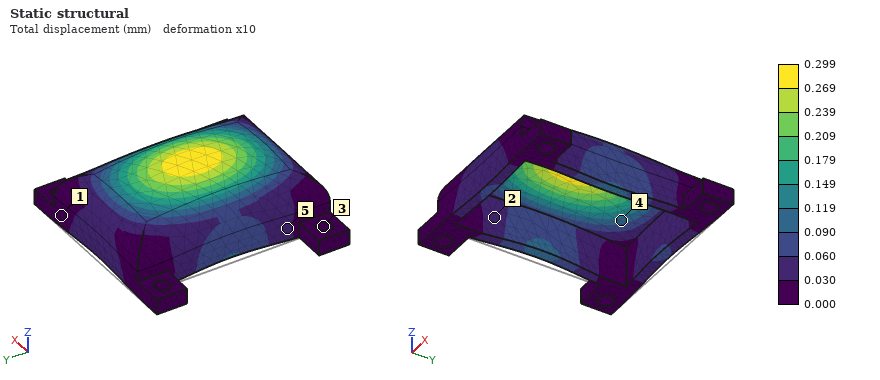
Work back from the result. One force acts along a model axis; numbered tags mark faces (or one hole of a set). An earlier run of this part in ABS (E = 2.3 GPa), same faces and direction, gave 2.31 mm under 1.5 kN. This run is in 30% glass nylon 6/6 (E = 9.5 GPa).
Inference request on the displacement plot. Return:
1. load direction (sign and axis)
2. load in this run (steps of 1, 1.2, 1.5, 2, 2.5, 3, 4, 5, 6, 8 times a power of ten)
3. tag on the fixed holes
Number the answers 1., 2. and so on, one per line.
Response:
1. +Z
2. 800 N
3. 3
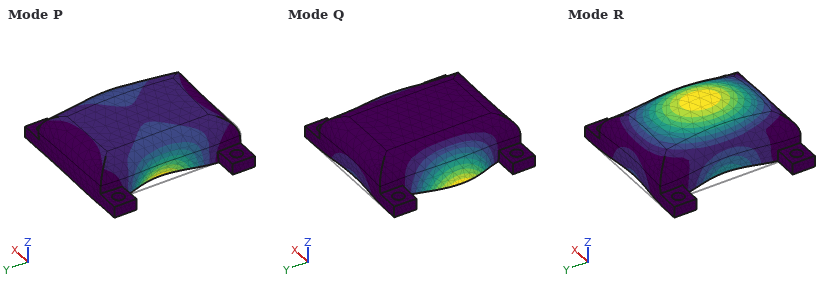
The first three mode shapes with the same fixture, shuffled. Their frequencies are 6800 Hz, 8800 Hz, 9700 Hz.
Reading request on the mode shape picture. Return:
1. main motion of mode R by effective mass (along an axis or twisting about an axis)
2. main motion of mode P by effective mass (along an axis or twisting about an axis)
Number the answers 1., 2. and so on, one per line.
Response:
1. along Z
2. along X
